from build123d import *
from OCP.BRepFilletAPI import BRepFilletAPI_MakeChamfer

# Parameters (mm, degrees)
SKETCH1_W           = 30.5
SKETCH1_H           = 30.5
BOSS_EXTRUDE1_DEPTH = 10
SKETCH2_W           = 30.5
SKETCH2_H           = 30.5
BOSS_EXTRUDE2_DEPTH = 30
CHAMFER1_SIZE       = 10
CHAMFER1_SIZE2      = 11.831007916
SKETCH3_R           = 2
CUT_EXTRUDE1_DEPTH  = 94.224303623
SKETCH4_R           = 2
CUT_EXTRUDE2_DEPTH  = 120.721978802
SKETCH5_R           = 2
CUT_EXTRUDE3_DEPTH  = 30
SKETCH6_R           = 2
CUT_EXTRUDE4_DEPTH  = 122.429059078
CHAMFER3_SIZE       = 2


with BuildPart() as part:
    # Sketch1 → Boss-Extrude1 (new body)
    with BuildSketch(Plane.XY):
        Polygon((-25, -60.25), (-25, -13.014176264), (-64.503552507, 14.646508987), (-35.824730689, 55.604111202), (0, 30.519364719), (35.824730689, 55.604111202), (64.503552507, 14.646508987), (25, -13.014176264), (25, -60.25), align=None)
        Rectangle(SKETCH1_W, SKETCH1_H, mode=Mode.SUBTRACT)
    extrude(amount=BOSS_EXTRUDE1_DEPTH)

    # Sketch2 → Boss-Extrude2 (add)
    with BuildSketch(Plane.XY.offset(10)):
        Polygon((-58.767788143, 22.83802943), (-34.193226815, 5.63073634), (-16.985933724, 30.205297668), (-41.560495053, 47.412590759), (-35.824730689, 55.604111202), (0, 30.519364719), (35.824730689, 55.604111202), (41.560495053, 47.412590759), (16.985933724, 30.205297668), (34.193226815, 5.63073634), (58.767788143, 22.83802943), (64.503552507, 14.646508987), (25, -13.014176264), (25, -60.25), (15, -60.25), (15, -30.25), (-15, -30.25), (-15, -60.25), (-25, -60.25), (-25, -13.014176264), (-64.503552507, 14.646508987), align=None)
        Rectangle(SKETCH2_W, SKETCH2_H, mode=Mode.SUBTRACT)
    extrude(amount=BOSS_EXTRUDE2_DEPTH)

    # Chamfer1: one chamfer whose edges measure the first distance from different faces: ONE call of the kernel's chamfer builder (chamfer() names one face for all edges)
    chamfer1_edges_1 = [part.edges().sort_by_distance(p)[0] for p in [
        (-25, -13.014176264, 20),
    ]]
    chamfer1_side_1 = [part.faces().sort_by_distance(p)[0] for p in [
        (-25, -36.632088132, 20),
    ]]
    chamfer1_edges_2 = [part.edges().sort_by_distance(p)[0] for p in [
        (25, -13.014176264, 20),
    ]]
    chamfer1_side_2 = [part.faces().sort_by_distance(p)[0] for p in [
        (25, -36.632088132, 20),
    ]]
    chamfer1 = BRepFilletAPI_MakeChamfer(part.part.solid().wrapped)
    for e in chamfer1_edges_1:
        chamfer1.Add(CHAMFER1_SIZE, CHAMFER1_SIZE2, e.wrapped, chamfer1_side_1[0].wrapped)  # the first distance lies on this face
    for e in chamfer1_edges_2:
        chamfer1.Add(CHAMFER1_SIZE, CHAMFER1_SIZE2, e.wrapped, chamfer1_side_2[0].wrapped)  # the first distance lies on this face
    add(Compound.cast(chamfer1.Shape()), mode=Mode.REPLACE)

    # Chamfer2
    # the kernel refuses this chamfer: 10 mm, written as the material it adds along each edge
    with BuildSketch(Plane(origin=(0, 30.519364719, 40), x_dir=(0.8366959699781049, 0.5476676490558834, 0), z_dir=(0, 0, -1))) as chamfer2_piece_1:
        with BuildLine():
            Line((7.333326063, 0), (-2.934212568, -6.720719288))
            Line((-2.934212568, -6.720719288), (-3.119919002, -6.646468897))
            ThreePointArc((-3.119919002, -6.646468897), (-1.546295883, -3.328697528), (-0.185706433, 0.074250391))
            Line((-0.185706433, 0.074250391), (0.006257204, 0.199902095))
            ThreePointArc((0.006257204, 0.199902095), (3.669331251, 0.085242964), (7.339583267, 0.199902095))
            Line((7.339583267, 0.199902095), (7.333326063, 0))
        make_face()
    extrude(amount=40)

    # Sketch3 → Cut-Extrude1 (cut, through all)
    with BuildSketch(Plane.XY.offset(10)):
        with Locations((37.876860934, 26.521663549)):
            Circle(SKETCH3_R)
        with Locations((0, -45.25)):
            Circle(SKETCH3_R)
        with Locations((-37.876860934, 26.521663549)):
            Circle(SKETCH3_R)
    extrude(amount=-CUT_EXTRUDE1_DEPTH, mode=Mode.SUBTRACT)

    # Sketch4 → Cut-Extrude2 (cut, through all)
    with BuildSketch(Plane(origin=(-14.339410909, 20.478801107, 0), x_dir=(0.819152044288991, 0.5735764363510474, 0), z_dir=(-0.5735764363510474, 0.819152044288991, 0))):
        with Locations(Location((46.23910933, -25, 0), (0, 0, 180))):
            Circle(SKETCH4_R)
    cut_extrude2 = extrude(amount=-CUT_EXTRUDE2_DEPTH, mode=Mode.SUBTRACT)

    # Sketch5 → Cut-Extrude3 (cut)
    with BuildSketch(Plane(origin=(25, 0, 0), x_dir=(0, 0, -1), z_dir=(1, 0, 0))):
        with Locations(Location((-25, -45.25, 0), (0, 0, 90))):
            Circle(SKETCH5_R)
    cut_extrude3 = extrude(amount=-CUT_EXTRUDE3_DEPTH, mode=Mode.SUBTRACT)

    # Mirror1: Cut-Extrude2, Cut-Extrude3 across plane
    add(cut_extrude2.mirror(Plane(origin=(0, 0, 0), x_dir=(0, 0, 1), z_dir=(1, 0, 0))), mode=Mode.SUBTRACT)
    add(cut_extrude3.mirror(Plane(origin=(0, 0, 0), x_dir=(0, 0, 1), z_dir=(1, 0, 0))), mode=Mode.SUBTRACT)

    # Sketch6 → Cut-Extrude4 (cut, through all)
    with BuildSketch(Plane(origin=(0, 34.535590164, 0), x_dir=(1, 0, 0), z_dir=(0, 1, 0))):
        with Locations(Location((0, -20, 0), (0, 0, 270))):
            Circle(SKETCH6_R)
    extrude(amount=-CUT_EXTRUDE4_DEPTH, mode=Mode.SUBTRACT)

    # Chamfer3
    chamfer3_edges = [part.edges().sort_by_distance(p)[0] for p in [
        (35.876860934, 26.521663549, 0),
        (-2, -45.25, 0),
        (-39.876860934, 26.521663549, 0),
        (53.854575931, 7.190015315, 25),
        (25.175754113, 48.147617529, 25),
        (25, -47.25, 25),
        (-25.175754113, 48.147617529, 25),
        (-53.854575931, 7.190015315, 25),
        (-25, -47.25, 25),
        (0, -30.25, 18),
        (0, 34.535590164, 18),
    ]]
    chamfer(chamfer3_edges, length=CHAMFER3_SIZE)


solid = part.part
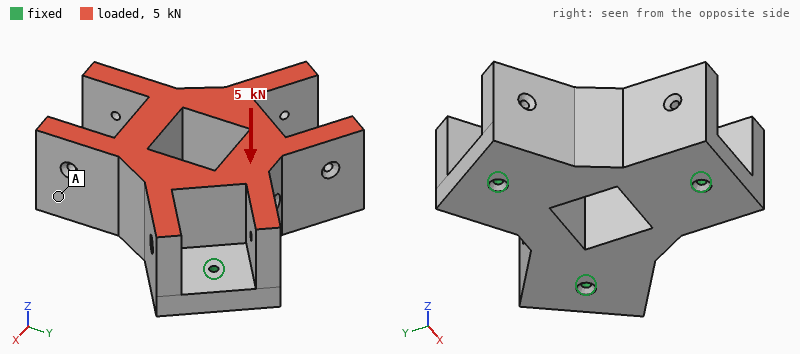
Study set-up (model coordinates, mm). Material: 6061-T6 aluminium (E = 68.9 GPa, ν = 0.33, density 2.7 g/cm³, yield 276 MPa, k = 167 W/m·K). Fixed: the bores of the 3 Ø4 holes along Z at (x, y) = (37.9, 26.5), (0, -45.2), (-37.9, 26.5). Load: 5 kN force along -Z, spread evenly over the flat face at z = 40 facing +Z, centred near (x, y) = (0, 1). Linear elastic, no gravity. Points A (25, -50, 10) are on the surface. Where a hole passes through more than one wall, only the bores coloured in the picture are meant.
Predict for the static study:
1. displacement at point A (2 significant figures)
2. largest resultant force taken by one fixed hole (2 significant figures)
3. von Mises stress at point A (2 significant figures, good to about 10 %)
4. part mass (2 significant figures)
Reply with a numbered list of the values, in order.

1. 7.8 µm
2. 1.8 kN
3. 3.1 MPa
4. 560 g
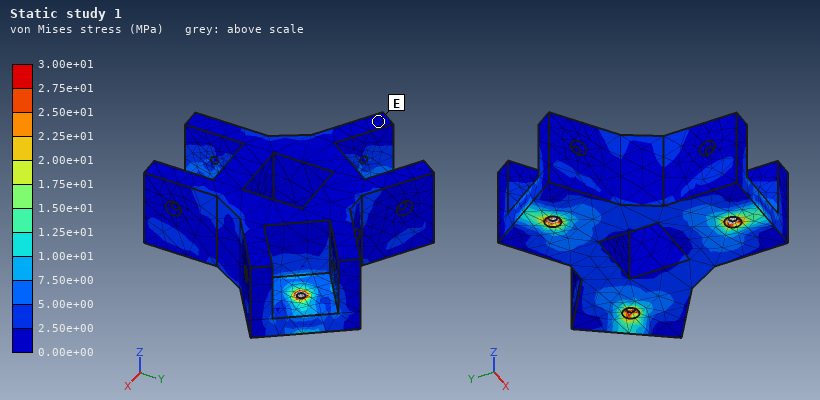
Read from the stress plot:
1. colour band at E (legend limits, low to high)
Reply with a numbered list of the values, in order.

1. 0.00e+00 to 2.50e+00 MPa
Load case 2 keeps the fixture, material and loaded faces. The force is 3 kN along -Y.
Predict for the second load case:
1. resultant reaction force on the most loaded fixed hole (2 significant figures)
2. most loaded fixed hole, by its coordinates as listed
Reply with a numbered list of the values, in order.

1. 1.9 kN
2. (0, -45.2)
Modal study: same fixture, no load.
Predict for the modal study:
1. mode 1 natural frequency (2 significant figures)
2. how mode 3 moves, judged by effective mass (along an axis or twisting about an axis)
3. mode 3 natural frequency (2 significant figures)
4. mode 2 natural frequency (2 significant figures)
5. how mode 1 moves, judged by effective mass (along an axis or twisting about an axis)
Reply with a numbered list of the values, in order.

1. 4900 Hz
2. along Z
3. 5700 Hz
4. 5300 Hz
5. along X
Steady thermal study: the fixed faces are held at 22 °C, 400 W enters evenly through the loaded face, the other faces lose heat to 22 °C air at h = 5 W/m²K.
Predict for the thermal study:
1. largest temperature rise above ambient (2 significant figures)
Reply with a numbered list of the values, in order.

1. 55 K
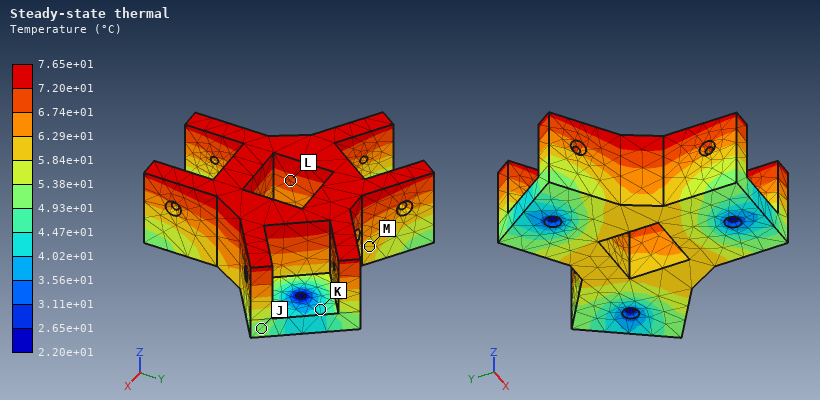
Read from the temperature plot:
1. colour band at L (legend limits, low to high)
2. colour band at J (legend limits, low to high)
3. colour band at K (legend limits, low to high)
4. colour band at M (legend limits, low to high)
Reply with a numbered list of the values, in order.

1. 6.74e+01 to 7.20e+01 °C
2. 4.93e+01 to 5.38e+01 °C
3. 4.02e+01 to 4.47e+01 °C
4. 5.84e+01 to 6.29e+01 °C
